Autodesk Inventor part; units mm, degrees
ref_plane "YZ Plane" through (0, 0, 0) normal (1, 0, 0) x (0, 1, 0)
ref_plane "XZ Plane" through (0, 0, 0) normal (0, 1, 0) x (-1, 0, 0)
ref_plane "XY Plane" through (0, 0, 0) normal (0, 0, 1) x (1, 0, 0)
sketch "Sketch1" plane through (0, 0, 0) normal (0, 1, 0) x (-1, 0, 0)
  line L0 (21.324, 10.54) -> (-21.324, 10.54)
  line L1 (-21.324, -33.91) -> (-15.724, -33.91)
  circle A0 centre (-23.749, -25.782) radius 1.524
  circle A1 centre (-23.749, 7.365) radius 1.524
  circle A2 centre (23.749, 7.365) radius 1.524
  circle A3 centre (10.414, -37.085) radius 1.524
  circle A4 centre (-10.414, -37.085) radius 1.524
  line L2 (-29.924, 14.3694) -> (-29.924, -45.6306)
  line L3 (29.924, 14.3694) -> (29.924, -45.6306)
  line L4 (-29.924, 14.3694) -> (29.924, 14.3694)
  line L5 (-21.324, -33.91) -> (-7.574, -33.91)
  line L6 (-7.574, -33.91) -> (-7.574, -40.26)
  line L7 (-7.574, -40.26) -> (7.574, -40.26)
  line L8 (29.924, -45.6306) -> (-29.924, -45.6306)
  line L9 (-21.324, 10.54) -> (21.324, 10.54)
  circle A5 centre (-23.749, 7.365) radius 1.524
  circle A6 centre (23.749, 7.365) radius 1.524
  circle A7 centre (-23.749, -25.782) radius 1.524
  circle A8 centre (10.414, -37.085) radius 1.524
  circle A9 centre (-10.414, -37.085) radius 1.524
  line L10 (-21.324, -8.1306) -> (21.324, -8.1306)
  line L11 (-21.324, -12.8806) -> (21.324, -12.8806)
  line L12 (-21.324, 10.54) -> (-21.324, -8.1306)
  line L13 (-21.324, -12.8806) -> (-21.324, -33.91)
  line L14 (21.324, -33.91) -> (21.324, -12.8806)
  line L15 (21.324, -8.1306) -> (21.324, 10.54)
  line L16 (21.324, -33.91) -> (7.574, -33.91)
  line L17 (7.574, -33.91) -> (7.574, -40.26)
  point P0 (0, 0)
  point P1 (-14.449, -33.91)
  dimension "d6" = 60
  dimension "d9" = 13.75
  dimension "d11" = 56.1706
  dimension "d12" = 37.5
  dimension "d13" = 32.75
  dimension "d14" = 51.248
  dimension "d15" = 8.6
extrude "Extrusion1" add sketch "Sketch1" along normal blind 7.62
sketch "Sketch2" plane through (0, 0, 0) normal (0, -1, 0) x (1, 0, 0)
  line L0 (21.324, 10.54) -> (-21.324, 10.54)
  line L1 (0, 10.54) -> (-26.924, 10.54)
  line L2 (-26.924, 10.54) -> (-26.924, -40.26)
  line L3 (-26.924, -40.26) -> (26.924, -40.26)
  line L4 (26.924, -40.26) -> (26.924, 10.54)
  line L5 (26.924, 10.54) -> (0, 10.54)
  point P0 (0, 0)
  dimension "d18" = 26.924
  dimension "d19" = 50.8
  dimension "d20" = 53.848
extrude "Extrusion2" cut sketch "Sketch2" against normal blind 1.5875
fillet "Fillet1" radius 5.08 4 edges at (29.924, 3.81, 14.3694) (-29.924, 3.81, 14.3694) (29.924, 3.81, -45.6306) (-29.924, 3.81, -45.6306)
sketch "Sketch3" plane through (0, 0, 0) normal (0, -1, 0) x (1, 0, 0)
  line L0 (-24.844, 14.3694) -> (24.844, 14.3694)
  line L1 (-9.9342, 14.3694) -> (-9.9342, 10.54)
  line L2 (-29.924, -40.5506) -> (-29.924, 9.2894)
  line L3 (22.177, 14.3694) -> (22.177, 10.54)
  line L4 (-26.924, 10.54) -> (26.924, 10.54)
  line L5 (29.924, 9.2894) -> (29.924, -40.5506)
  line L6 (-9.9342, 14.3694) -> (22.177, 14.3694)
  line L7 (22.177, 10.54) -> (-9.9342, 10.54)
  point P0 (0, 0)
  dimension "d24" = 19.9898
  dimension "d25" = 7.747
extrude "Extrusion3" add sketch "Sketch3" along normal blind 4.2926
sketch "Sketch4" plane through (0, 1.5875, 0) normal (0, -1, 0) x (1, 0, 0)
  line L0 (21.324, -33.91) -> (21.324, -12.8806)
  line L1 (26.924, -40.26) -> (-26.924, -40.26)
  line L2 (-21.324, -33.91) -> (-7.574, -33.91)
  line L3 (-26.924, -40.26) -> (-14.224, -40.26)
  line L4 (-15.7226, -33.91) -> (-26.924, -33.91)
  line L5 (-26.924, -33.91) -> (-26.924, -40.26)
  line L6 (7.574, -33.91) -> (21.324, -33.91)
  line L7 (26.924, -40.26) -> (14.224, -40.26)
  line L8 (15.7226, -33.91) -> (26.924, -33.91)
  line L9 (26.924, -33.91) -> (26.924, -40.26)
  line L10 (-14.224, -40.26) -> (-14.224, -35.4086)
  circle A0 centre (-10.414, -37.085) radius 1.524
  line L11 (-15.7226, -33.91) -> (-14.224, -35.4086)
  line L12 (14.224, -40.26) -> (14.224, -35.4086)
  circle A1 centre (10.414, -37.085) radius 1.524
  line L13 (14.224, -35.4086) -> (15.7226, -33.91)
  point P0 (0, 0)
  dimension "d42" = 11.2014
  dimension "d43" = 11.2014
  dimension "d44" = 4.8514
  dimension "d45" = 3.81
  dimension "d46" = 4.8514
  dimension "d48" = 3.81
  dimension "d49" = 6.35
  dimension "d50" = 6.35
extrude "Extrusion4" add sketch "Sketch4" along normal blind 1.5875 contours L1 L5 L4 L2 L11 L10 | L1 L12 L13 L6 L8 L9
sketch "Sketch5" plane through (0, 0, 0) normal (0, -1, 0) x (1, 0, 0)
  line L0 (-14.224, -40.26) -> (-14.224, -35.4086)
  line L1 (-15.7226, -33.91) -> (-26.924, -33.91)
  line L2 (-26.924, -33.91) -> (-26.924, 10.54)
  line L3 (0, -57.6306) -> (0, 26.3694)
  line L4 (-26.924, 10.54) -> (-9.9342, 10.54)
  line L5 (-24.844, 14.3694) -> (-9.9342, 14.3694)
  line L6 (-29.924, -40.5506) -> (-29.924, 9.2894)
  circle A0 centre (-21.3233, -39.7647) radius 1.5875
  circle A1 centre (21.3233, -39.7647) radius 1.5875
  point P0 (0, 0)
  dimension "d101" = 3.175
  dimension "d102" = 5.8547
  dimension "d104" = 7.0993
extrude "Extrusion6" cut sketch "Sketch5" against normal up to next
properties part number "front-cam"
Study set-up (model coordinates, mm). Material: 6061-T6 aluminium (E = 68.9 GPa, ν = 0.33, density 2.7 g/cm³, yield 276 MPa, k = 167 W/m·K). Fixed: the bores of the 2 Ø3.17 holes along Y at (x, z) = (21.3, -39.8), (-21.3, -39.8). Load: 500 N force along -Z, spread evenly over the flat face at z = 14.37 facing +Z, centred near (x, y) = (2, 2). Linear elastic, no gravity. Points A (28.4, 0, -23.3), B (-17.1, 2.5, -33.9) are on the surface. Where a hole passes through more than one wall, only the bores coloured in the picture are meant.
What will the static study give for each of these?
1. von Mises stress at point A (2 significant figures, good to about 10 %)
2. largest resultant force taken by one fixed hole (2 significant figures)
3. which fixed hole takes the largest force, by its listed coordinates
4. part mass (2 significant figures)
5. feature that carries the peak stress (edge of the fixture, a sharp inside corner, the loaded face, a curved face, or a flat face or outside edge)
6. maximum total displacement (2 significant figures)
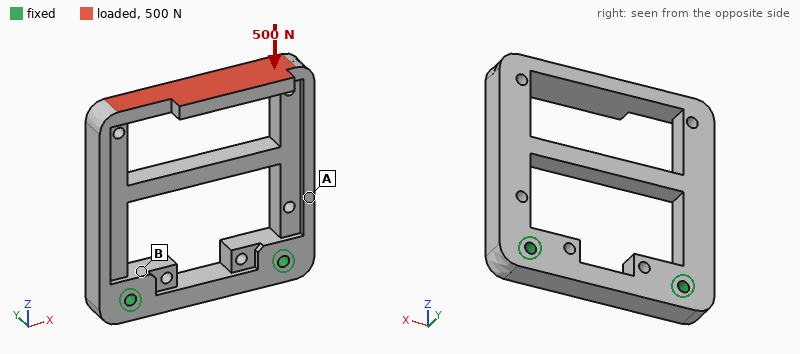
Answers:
17 MPa
270 N
(21.3, -39.8)
34 g
a curved face
0.11 mm
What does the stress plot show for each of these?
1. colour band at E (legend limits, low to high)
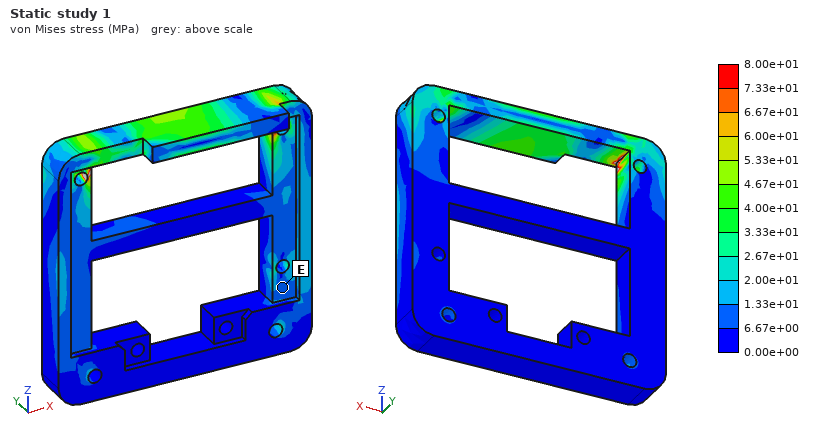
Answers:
6.67e+00 to 1.33e+01 MPa
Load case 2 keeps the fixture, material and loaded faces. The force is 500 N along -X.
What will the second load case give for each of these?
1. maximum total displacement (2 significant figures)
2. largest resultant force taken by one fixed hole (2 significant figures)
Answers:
0.27 mm
450 N
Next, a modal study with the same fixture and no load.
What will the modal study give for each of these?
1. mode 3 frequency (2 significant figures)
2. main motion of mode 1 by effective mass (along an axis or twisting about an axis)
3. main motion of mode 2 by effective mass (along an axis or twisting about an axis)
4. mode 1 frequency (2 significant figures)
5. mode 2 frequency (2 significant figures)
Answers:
2600 Hz
along Y
along X
1300 Hz
2200 Hz
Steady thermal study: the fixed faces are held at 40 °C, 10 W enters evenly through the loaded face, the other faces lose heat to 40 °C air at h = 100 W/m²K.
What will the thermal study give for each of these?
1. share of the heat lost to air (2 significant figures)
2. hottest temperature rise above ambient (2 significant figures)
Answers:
53 %
25 K
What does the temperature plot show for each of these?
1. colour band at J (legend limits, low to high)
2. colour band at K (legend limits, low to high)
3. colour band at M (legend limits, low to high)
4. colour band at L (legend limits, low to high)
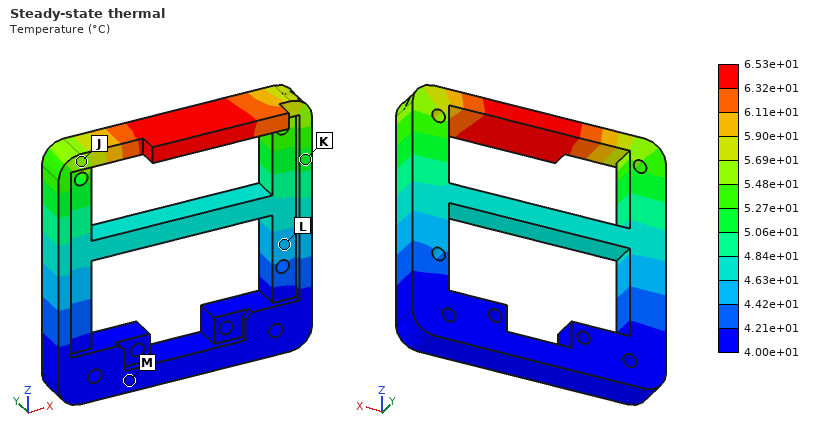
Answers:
5.48e+01 to 5.69e+01 °C
5.06e+01 to 5.27e+01 °C
4.00e+01 to 4.21e+01 °C
4.42e+01 to 4.63e+01 °C
